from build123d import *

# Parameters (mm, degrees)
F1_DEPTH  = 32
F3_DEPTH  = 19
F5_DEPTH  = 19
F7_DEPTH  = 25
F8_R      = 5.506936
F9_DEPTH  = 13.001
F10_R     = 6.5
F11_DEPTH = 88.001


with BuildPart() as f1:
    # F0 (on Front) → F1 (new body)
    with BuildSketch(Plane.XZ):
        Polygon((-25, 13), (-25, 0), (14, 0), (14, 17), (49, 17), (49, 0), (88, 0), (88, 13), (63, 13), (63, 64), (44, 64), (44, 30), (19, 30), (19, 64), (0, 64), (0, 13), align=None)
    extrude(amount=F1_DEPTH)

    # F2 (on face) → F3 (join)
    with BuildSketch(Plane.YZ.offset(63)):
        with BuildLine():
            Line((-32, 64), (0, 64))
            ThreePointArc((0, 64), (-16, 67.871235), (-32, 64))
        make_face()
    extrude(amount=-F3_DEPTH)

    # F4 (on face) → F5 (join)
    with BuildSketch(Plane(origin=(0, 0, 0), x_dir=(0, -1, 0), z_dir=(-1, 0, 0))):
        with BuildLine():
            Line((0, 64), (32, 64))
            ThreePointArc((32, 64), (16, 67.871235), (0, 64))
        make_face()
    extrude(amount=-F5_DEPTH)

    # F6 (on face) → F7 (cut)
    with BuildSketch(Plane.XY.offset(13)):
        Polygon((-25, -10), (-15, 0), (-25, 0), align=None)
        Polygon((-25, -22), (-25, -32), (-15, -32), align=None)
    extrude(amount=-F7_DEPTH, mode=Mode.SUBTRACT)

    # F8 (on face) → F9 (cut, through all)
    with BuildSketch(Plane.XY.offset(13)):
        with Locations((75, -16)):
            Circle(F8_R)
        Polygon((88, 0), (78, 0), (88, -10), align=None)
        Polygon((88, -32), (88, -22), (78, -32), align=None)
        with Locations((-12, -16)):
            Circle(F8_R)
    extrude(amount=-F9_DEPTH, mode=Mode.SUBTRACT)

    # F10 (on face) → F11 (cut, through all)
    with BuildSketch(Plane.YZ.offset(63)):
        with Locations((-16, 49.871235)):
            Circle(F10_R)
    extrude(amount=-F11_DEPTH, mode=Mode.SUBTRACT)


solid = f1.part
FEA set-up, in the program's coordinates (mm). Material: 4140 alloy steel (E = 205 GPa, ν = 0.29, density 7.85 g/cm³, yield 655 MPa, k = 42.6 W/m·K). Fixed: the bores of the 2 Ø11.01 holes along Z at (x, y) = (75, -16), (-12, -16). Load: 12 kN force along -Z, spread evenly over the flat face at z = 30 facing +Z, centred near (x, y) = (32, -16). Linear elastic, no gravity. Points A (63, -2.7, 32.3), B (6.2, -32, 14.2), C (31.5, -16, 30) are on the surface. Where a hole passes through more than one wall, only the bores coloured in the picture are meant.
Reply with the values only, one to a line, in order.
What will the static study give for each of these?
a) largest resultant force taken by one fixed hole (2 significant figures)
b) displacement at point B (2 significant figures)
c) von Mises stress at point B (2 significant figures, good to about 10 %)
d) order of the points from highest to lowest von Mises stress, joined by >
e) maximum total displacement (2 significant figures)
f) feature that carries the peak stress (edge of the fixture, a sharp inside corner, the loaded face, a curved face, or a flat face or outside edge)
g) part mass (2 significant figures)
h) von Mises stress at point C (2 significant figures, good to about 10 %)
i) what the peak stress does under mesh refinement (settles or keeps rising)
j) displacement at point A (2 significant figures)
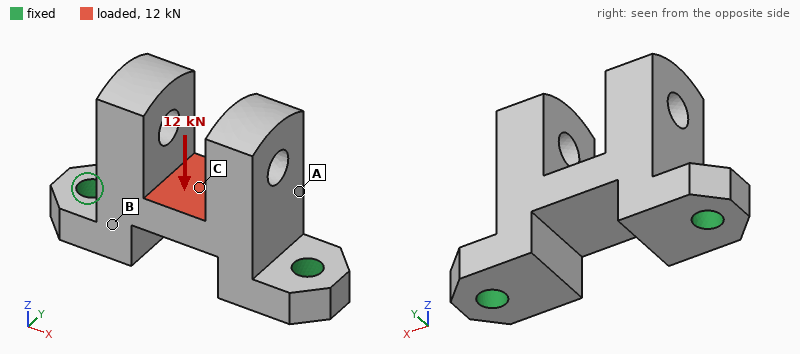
8.9 kN
5.7 µm
32 MPa
C > B > A
20 µm
edge of the fixture
760 g
58 MPa
keeps rising
5.5 µm
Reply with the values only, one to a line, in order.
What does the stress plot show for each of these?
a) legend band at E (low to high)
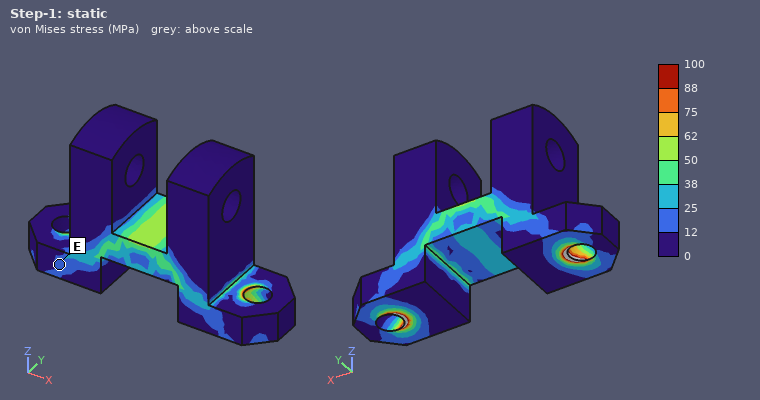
12 to 25 MPa
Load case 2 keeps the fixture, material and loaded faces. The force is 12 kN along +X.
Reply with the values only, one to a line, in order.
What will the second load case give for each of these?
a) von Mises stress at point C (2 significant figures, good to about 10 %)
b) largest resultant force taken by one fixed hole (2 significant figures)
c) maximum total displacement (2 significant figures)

26 MPa
7.0 kN
11 µm
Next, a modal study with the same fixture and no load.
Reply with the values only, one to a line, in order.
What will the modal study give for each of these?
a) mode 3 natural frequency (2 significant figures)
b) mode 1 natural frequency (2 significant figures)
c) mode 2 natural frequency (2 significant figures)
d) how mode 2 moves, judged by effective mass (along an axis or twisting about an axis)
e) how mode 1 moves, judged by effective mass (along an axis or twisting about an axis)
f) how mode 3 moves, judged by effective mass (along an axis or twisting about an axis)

5100 Hz
2600 Hz
4300 Hz
twisting about Z
along Y
along X
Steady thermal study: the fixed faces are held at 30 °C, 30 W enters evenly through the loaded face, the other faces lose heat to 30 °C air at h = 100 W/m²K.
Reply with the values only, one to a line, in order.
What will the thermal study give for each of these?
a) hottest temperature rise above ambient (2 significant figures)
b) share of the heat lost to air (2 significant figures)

24 K
54 %
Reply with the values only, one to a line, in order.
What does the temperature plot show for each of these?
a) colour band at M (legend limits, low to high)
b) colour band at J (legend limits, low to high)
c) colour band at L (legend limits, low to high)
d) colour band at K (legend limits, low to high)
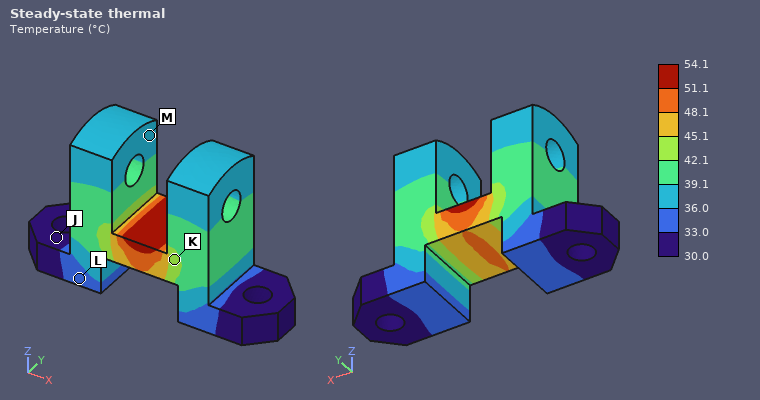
36.0 to 39.1 °C
30.0 to 33.0 °C
33.0 to 36.0 °C
42.1 to 45.1 °C
